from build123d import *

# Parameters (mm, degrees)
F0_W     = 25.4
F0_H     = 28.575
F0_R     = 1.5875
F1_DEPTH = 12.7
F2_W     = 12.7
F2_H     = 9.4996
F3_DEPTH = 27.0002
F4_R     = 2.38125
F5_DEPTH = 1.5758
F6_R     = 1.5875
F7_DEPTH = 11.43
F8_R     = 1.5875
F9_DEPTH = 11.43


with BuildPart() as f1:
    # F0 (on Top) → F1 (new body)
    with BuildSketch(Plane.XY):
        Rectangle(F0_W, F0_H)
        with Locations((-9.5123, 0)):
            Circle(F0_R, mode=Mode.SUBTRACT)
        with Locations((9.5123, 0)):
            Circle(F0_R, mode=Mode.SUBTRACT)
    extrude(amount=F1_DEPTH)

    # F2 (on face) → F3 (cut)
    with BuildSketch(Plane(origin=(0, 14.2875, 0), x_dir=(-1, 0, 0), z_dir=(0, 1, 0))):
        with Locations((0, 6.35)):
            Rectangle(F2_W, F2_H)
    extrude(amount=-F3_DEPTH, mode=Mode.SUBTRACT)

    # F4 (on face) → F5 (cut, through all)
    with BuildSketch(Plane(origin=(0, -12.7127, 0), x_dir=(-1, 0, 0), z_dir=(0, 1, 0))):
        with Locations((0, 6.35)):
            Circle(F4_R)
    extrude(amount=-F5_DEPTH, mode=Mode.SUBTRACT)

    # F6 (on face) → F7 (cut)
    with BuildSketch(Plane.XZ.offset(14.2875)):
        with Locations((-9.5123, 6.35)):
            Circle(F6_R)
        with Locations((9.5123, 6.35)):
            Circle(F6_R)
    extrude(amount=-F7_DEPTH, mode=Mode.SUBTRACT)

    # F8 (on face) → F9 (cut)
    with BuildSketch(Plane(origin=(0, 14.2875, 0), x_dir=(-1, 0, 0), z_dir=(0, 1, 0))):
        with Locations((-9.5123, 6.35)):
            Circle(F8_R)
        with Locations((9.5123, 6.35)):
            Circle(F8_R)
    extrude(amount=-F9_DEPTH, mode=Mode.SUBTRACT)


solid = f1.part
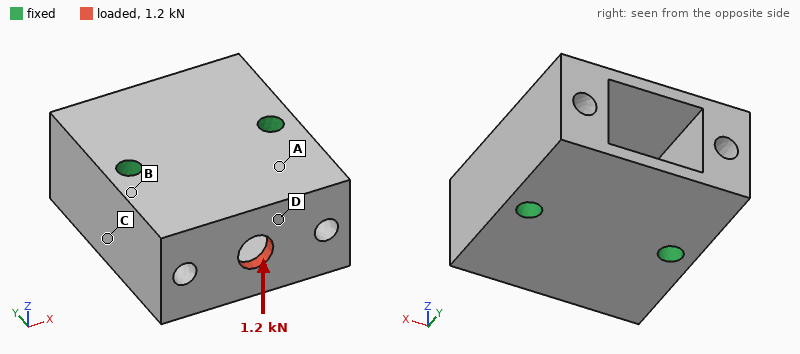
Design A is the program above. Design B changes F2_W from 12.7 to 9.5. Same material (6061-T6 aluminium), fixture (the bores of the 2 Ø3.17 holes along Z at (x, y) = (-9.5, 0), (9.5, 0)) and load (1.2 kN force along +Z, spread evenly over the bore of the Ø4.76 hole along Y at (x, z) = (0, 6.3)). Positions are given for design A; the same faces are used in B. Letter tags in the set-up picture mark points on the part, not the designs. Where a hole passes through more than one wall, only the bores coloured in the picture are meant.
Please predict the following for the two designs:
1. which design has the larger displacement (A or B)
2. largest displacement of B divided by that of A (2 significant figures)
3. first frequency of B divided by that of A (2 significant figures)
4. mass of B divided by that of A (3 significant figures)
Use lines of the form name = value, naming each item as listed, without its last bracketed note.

which design has the larger displacement = A
largest displacement of B divided by that of A = 0.79
first frequency of B divided by that of A = 1.0
mass of B divided by that of A = 1.15
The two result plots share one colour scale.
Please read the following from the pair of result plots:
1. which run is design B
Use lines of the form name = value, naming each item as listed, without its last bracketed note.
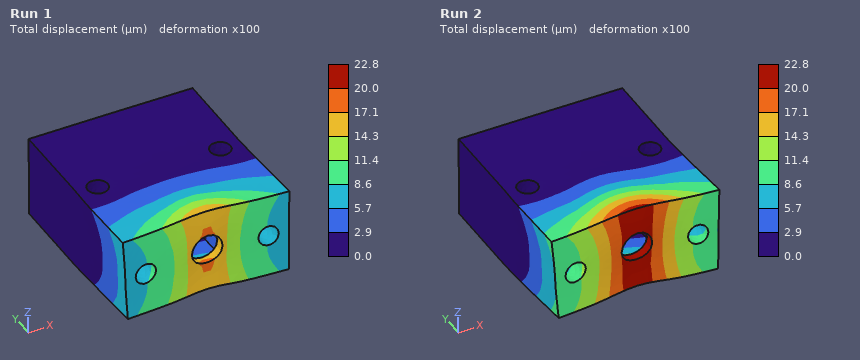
which run is design B = Run 1
